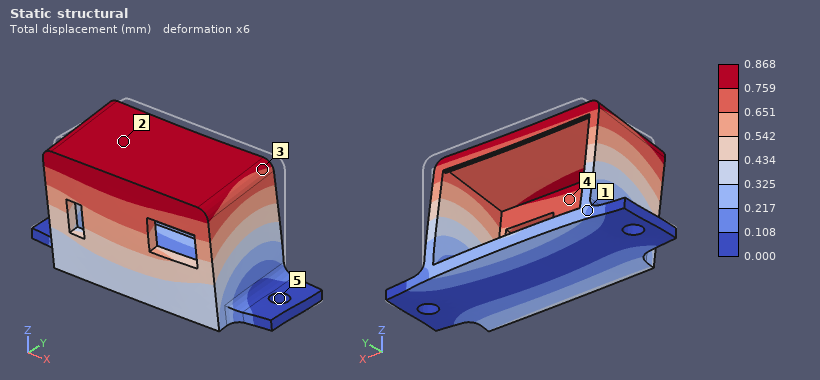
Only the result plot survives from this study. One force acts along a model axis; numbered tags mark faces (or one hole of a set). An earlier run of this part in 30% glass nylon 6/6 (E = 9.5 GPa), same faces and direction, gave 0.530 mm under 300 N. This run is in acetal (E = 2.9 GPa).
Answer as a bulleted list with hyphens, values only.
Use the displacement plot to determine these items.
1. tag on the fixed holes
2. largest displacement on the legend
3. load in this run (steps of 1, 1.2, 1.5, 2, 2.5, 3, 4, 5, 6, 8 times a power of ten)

- 5
- 0.868 mm
- 150 N
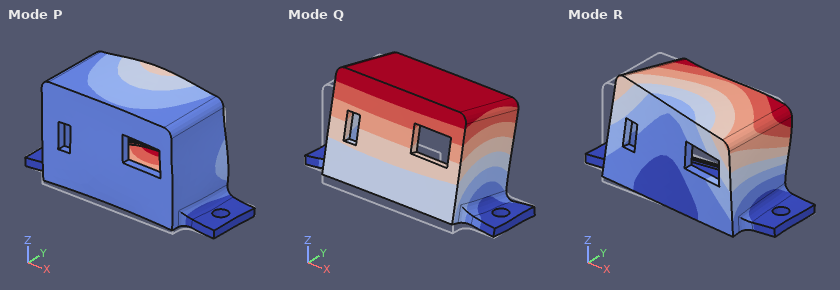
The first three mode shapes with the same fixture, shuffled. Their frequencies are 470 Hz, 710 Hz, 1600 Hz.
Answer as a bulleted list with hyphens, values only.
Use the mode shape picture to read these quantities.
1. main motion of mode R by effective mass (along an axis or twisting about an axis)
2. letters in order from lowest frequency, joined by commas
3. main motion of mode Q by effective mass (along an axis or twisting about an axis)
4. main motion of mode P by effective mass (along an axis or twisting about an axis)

- along X
- Q, R, P
- along Y
- along Z
